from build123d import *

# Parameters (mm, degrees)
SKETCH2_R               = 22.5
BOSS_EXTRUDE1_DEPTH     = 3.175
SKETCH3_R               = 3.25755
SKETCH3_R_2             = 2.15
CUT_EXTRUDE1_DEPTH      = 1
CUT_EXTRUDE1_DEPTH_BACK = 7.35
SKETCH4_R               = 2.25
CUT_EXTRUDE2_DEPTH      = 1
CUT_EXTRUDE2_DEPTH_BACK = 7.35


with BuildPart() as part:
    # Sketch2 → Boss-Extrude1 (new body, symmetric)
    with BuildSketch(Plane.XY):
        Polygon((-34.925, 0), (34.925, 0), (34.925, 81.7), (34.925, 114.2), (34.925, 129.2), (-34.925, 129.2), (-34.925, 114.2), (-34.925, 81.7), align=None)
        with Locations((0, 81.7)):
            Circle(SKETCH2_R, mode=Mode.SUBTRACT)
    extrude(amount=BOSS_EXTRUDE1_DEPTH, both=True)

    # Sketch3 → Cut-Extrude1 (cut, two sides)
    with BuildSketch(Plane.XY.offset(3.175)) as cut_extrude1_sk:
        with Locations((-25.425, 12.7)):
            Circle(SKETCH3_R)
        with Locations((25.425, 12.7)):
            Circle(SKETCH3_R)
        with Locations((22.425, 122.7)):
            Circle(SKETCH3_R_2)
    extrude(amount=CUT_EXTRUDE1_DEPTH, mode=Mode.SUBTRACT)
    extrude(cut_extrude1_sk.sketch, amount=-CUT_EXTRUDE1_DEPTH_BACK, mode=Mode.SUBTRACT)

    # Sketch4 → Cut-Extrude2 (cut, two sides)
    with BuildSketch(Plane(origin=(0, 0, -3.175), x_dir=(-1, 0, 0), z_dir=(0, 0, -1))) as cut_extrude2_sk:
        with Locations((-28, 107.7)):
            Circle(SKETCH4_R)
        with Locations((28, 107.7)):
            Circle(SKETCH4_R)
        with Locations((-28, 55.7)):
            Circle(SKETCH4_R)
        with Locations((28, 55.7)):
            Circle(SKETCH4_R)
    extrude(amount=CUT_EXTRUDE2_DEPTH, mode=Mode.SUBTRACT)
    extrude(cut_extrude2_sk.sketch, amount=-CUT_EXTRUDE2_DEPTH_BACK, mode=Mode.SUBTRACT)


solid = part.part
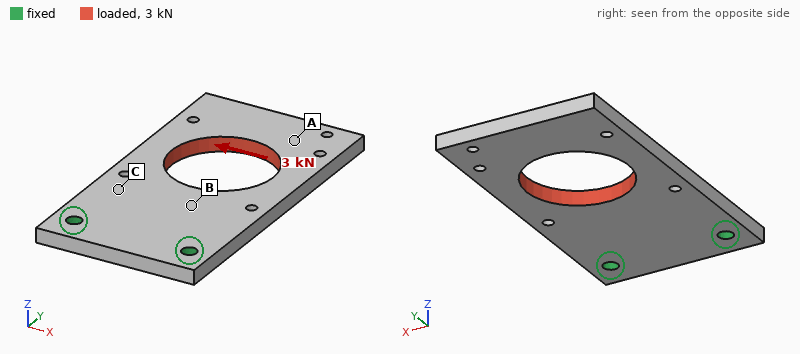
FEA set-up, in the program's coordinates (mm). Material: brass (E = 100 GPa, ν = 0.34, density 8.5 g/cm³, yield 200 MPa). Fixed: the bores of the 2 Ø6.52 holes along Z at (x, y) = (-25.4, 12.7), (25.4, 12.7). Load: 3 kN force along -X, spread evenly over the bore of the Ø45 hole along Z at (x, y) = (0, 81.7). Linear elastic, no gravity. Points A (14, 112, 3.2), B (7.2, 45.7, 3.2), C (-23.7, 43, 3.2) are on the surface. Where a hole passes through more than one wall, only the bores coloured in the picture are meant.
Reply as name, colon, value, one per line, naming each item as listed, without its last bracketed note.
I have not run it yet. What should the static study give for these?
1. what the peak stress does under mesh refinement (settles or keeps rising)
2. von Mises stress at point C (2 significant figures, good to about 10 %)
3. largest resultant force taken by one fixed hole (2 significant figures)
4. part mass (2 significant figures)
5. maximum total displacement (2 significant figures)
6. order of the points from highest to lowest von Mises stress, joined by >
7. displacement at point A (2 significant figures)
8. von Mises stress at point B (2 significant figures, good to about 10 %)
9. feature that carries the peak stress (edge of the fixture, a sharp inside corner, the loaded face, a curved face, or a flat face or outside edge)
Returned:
what the peak stress does under mesh refinement: keeps rising
von Mises stress at point C: 13 MPa
largest resultant force taken by one fixed hole: 4.1 kN
part mass: 390 g
maximum total displacement: 0.10 mm
order of the points from highest to lowest von Mises stress, joined by >: B > C > A
displacement at point A: 0.090 mm
von Mises stress at point B: 26 MPa
feature that carries the peak stress: edge of the fixture
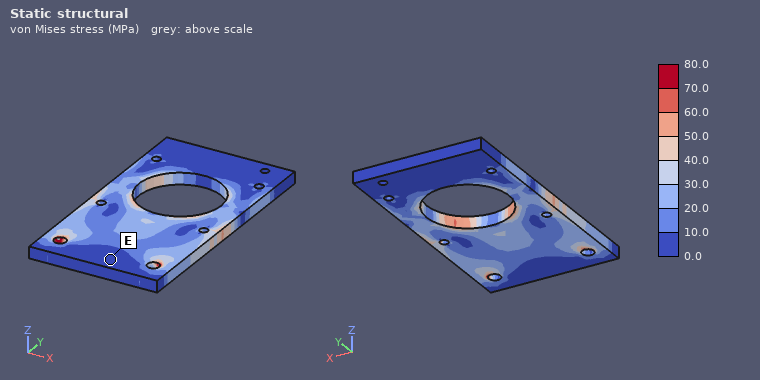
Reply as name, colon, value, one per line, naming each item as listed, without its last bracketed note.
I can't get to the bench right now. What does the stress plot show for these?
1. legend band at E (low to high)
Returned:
legend band at E: 0.0 to 10.0 MPa
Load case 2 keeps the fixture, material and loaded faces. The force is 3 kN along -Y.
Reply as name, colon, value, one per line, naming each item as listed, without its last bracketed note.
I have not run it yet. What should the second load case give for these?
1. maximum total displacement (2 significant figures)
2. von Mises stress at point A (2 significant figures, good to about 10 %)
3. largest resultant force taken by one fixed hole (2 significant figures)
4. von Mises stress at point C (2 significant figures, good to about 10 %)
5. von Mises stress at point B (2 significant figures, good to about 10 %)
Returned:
maximum total displacement: 12 µm
von Mises stress at point A: 4.6 MPa
largest resultant force taken by one fixed hole: 1.5 kN
von Mises stress at point C: 8.2 MPa
von Mises stress at point B: 3.5 MPa
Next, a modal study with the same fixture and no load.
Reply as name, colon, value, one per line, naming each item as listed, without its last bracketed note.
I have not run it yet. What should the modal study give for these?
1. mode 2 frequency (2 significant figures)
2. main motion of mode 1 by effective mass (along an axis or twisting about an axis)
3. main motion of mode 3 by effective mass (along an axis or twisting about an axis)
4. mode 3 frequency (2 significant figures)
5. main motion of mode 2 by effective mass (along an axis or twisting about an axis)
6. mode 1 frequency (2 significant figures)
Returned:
mode 2 frequency: 830 Hz
main motion of mode 1 by effective mass: along Z
main motion of mode 3 by effective mass: along Z
mode 3 frequency: 1400 Hz
main motion of mode 2 by effective mass: twisting about Y
mode 1 frequency: 260 Hz
